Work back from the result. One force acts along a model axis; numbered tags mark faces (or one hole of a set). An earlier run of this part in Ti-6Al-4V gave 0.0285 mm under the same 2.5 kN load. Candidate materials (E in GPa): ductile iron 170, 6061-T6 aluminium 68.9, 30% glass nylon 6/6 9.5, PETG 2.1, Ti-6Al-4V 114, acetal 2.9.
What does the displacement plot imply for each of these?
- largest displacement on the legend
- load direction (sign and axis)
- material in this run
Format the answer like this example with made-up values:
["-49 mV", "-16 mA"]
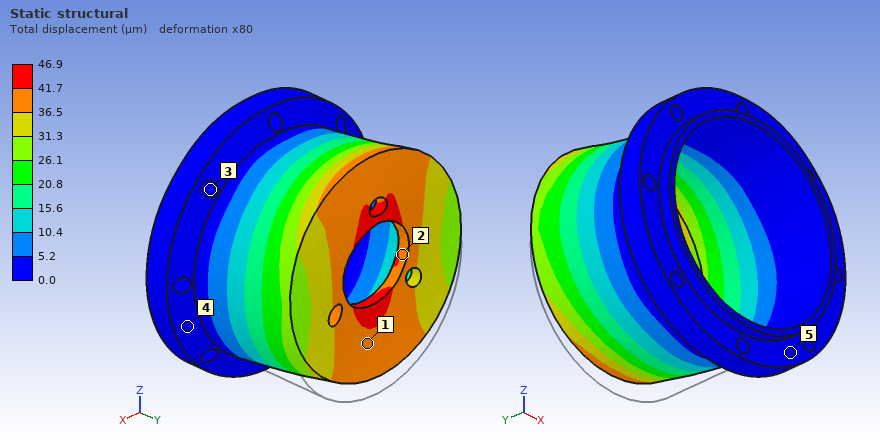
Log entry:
["46.9 µm", "+Z", "6061-T6 aluminium"]
